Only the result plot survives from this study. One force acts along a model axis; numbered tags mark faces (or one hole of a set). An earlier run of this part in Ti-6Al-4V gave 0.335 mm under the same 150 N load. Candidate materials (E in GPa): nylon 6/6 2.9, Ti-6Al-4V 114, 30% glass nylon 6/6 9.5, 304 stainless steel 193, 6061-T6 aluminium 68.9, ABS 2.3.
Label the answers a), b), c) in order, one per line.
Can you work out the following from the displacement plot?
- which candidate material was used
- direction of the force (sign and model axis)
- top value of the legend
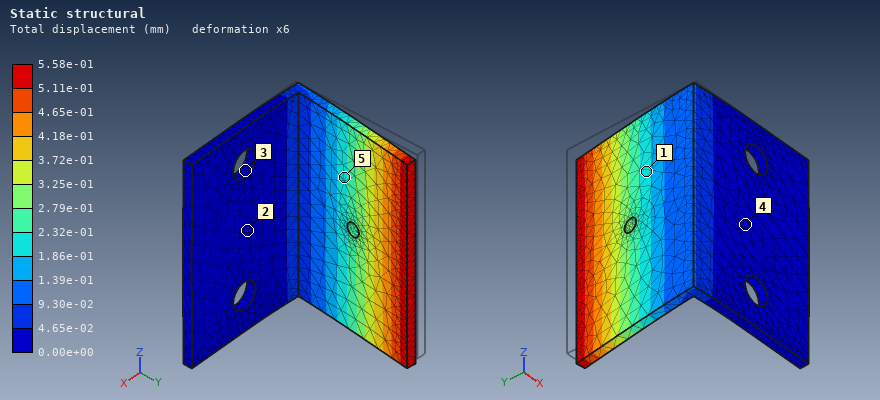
a) 6061-T6 aluminium
b) +X
c) 5.58e-01 mm
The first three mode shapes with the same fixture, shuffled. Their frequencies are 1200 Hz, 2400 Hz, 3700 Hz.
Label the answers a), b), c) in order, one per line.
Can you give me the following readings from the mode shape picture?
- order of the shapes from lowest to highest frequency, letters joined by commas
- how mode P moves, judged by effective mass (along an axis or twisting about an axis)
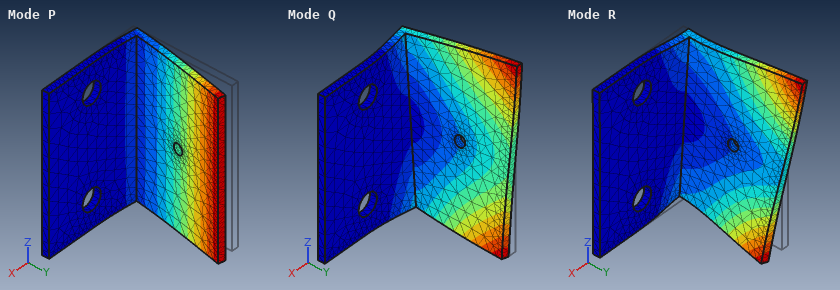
a) P, Q, R
b) along X
